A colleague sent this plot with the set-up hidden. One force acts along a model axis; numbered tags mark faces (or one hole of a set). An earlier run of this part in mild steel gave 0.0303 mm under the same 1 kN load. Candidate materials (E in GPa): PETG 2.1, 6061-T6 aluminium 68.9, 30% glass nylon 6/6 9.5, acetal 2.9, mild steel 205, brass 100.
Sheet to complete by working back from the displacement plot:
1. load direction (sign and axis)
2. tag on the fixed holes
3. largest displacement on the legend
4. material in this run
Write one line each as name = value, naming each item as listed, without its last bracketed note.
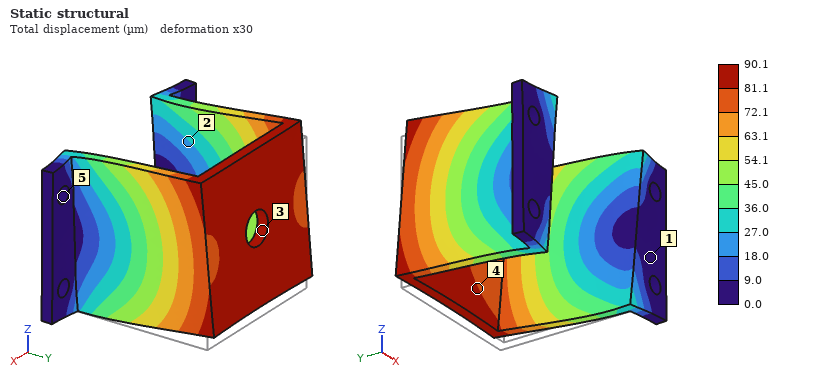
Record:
load direction = +Z
tag on the fixed holes = 5
largest displacement on the legend = 90.1 µm
material in this run = 6061-T6 aluminium
